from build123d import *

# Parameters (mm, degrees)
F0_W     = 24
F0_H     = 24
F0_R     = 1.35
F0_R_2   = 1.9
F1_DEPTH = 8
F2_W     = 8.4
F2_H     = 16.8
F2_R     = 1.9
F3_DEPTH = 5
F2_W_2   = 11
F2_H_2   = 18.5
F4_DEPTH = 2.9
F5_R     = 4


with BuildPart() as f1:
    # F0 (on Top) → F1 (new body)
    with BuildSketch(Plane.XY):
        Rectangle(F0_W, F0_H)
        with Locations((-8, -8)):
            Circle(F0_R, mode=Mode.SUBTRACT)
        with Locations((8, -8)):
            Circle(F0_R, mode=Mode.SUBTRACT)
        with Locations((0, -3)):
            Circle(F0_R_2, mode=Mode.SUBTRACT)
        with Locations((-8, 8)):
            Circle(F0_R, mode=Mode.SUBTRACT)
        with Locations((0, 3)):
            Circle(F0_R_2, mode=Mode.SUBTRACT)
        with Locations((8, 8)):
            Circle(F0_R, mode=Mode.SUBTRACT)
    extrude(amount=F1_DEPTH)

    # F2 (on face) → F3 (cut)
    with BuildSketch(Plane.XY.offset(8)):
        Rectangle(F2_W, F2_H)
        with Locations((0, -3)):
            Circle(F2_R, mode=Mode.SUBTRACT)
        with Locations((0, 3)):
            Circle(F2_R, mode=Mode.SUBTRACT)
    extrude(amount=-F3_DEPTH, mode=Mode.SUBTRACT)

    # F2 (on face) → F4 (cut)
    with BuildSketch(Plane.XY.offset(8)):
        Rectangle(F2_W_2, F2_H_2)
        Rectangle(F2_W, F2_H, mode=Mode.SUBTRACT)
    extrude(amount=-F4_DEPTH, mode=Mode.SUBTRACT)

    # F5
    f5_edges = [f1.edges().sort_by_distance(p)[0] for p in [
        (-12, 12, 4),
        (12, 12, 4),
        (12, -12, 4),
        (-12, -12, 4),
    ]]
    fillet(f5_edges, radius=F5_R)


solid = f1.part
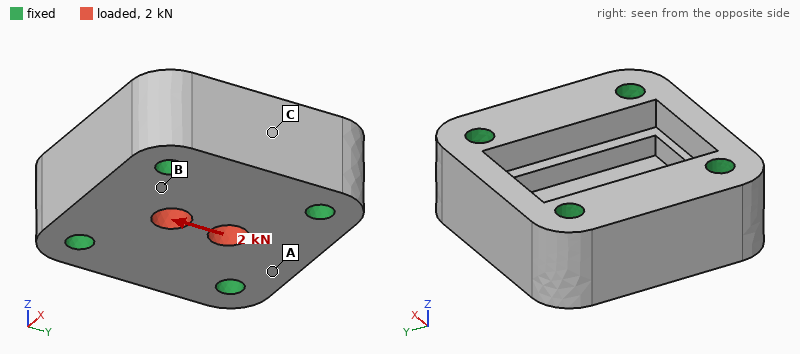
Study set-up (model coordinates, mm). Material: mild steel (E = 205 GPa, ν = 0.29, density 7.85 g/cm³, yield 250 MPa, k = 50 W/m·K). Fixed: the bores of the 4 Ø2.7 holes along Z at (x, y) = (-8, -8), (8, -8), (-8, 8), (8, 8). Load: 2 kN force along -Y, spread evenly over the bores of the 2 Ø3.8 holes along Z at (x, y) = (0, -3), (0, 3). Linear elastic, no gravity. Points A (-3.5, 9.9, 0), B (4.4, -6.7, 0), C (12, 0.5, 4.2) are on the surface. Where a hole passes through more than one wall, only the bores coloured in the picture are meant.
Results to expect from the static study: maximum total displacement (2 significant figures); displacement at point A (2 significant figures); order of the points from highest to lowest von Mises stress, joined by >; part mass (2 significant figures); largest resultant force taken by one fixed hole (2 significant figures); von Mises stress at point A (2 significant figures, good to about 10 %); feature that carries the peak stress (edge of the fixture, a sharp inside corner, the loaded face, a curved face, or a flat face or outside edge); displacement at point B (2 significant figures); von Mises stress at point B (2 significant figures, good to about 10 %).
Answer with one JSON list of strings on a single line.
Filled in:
["2.0 µm", "0.57 µm", "B > A > C", "26 g", "550 N", "14 MPa", "the loaded face", "0.49 µm", "24 MPa"]
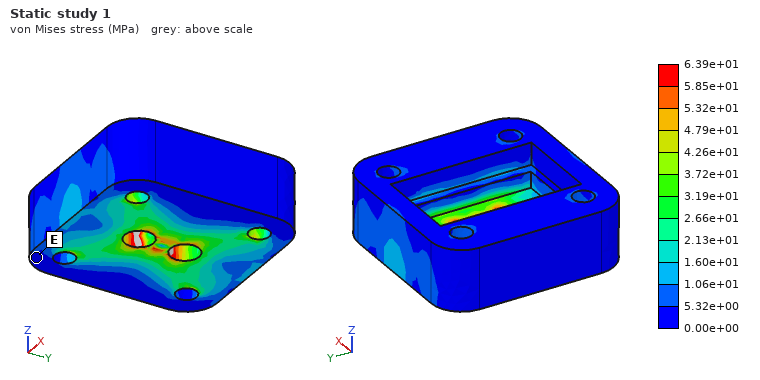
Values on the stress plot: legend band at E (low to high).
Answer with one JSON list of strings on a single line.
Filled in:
["0.00e+00 to 5.32e+00 MPa"]
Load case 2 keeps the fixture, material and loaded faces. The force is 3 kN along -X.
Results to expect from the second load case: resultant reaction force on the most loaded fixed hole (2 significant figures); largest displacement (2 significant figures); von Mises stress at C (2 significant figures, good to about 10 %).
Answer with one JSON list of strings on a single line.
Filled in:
["800 N", "2.1 µm", "14 MPa"]
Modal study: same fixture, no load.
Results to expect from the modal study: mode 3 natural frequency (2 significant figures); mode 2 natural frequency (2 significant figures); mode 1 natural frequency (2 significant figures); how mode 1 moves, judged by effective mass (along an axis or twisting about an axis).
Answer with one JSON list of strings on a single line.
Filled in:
["83 kHz", "80 kHz", "72 kHz", "along Z"]
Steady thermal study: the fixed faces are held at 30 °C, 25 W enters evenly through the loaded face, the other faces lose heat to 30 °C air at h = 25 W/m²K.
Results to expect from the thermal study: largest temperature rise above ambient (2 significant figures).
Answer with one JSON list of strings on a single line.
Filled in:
["41 K"]
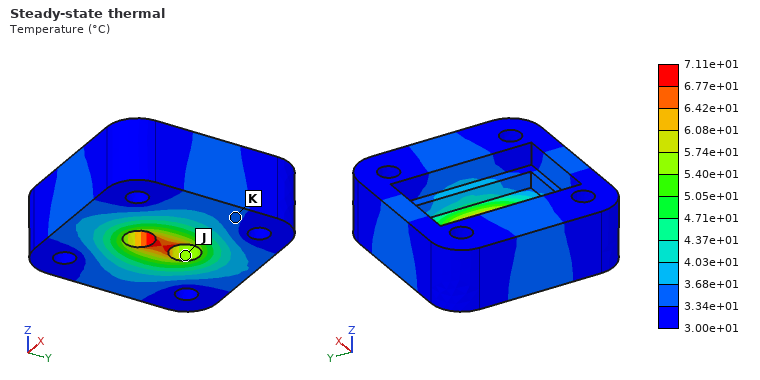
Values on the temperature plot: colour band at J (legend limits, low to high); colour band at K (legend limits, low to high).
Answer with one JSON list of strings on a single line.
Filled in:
["5.40e+01 to 5.74e+01 °C", "3.34e+01 to 3.68e+01 °C"]
